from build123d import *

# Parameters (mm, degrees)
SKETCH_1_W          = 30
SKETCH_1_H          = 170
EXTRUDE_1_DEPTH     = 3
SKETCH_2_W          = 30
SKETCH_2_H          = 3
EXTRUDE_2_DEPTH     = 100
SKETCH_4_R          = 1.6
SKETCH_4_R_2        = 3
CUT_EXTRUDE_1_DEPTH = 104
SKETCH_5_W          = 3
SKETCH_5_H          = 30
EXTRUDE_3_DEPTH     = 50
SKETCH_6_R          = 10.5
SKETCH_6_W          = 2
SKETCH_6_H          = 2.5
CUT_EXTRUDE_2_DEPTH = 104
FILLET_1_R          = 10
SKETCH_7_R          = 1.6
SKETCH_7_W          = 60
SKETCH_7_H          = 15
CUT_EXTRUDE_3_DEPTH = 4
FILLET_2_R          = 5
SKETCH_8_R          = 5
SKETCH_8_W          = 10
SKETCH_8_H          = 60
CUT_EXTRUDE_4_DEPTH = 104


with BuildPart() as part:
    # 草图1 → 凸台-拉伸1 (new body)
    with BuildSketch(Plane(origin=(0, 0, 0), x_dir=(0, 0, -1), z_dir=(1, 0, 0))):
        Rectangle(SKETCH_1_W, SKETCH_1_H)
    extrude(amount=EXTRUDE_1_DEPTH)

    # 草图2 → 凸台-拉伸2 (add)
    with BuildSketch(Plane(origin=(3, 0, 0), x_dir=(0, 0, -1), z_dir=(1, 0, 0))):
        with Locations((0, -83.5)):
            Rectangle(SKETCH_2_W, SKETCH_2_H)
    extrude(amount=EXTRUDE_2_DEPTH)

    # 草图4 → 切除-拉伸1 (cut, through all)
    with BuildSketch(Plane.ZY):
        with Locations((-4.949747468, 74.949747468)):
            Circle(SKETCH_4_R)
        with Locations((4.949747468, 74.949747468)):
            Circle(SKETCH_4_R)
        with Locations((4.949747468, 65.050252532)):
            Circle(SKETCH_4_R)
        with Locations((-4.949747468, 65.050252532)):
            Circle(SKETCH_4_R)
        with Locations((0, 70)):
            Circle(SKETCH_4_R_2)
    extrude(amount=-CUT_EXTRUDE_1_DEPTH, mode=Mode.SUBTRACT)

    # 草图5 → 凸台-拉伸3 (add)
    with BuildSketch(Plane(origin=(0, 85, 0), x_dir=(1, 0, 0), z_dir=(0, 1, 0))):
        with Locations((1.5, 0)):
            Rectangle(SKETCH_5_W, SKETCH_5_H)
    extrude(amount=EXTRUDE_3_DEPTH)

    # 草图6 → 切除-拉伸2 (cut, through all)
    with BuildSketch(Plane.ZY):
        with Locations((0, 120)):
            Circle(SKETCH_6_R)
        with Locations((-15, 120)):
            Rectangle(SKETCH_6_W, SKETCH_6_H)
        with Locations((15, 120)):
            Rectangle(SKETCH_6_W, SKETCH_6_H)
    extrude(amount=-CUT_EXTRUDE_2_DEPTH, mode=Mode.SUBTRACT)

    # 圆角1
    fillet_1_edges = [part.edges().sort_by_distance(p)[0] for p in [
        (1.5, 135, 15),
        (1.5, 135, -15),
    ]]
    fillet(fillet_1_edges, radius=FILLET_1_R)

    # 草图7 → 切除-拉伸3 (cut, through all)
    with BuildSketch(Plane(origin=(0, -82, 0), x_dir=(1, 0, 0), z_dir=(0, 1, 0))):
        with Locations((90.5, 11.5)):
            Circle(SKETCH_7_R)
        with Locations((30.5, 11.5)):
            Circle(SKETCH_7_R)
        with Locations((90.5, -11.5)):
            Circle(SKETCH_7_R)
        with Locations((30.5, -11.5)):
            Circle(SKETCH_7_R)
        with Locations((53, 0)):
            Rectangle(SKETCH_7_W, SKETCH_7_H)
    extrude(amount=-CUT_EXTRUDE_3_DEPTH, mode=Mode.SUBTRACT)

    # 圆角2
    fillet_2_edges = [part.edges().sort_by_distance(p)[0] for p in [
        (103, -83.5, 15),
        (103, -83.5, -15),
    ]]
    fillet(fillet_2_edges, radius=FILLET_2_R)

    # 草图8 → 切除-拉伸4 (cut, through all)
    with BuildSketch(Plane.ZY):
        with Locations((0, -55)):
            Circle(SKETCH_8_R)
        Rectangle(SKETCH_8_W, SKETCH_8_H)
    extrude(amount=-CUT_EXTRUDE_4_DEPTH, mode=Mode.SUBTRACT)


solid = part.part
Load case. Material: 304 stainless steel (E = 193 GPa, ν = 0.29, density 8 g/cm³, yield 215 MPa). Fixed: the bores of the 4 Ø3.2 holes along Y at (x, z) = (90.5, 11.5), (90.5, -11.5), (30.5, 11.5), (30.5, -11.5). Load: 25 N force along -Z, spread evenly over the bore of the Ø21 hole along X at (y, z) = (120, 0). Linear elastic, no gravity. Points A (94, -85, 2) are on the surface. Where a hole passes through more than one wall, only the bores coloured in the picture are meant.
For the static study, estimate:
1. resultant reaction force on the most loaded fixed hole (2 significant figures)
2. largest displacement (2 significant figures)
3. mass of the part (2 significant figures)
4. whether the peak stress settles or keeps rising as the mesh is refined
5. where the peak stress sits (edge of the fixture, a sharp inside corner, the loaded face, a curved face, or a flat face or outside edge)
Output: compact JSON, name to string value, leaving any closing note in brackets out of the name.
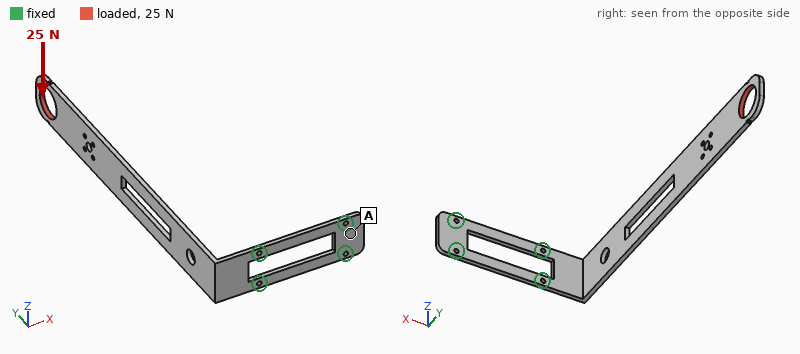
{"resultant reaction force on the most loaded fixed hole": "180 N", "largest displacement": "1.2 mm", "mass of the part": "180 g", "whether the peak stress settles or keeps rising as the mesh is refined": "keeps rising", "where the peak stress sits": "edge of the fixture"}
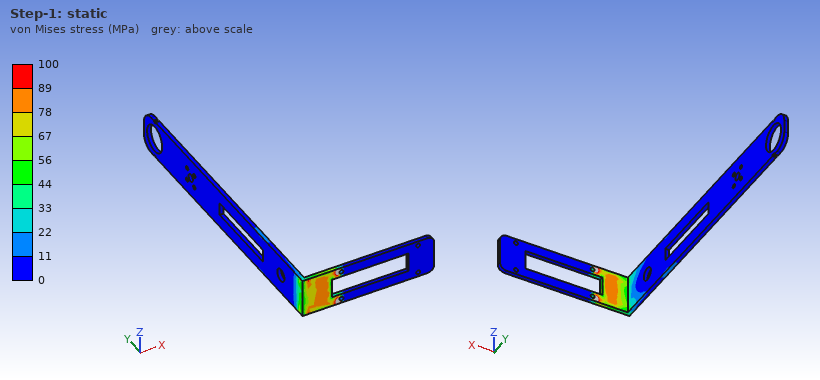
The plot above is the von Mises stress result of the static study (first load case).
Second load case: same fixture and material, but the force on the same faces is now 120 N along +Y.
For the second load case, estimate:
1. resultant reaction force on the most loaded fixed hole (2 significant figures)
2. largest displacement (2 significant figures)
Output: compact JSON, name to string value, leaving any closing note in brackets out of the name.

{"resultant reaction force on the most loaded fixed hole": "60 N", "largest displacement": "1.2 mm"}
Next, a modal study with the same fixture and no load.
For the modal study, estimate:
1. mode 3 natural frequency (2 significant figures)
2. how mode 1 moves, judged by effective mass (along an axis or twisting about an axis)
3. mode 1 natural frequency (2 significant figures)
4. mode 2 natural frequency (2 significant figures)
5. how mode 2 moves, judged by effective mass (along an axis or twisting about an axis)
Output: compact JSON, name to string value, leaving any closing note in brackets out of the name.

{"mode 3 natural frequency": "270 Hz", "how mode 1 moves, judged by effective mass": "along X", "mode 1 natural frequency": "42 Hz", "mode 2 natural frequency": "110 Hz", "how mode 2 moves, judged by effective mass": "along Z"}
